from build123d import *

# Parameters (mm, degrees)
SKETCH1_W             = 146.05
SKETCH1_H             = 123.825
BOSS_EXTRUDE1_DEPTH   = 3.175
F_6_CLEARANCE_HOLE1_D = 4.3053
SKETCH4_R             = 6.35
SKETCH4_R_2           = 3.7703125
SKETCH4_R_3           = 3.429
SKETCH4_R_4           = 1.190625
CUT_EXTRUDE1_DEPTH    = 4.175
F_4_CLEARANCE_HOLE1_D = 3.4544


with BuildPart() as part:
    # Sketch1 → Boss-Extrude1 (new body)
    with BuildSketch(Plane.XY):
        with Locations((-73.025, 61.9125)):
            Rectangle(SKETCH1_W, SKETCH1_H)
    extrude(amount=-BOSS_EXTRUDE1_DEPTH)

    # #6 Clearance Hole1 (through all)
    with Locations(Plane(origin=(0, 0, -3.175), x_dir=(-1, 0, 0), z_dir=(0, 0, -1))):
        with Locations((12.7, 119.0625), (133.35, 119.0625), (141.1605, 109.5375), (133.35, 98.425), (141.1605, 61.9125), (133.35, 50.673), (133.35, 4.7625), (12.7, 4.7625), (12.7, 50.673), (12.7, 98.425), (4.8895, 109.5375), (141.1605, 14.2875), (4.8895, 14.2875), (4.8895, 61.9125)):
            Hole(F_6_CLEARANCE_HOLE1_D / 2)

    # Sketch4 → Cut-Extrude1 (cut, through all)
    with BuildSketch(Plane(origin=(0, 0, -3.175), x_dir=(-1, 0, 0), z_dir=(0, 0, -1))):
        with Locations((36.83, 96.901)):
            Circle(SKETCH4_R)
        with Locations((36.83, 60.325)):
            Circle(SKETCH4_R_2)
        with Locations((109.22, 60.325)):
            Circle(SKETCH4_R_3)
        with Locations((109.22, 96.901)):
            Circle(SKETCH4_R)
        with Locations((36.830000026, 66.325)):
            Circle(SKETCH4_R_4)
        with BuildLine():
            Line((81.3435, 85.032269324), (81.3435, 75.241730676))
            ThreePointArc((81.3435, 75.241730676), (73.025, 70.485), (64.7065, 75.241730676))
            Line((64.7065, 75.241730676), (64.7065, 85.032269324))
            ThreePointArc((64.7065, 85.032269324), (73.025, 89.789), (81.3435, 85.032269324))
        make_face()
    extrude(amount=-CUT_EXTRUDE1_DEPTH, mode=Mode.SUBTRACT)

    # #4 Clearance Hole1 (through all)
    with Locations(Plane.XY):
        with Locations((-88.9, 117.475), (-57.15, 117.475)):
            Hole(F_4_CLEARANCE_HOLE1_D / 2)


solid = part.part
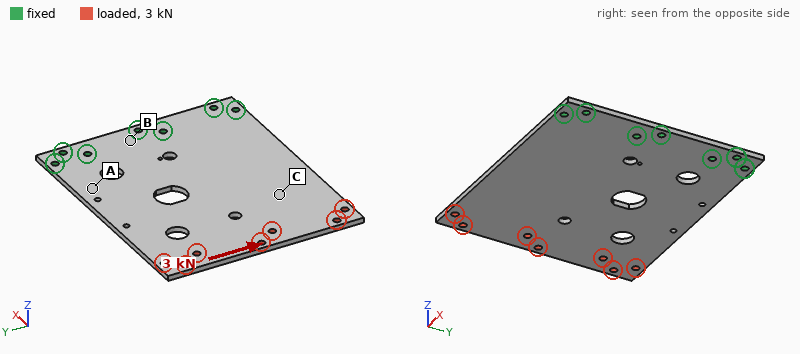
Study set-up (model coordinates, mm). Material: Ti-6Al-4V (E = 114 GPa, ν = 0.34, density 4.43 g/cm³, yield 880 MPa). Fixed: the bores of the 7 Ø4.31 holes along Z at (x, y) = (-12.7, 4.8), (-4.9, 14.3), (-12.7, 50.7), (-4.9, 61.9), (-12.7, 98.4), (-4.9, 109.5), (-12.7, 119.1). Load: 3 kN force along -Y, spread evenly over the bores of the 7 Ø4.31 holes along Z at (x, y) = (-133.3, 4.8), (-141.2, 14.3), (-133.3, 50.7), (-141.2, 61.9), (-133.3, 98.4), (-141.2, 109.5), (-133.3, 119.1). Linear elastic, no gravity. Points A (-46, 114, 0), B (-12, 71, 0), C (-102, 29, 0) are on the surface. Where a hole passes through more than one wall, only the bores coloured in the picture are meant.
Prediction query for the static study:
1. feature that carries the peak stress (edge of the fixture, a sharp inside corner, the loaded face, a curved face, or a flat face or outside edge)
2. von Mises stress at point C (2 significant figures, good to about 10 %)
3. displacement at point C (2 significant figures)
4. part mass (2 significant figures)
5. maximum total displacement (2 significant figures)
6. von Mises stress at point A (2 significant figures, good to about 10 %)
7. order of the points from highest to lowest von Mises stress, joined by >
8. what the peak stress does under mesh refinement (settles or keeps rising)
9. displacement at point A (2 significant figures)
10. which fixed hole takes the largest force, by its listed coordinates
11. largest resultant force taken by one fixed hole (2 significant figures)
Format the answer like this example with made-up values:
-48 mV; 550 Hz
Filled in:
edge of the fixture; 16 MPa; 46 µm; 240 g; 81 µm; 32 MPa; A > C > B; keeps rising; 17 µm; (-12.7, 4.8); 2.3 kN
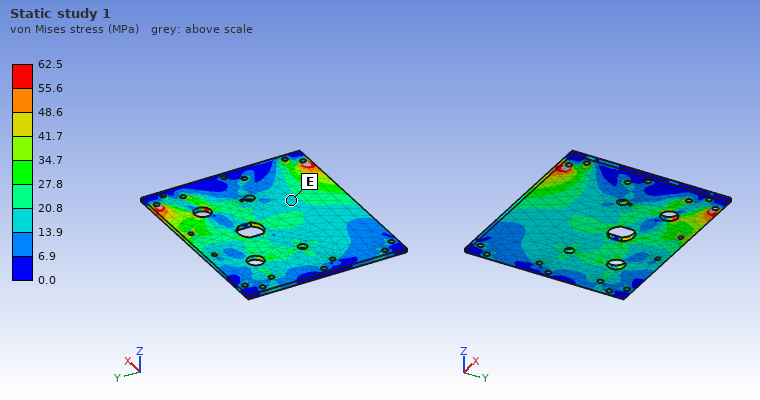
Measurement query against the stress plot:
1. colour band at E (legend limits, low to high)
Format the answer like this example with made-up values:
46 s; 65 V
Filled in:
13.9 to 20.8 MPa
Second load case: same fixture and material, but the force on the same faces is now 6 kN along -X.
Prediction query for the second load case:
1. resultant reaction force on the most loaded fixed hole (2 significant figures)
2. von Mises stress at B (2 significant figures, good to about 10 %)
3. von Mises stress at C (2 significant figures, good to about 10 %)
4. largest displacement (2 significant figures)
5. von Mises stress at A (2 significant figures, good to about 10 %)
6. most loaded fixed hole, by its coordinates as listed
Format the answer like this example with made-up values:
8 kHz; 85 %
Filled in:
1.3 kN; 10 MPa; 13 MPa; 30 µm; 23 MPa; (-12.7, 50.7)
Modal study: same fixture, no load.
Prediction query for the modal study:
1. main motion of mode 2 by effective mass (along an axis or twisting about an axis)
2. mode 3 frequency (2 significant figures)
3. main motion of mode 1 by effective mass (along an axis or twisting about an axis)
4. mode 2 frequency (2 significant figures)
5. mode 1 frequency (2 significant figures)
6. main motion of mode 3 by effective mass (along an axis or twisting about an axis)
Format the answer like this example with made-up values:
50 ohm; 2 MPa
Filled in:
twisting about X; 900 Hz; along Z; 380 Hz; 140 Hz; along Z
